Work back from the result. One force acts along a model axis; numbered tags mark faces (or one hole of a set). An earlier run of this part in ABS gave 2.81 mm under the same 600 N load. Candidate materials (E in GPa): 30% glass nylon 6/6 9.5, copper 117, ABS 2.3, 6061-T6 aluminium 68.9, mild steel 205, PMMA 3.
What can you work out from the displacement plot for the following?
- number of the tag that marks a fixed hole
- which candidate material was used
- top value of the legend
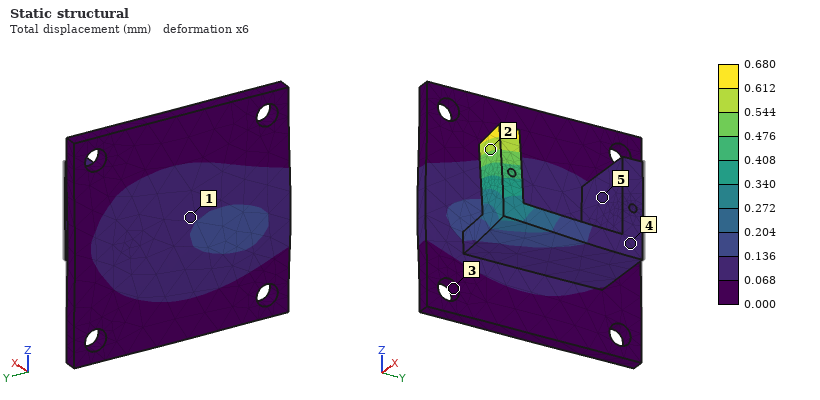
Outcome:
3
30% glass nylon 6/6
0.680 mm
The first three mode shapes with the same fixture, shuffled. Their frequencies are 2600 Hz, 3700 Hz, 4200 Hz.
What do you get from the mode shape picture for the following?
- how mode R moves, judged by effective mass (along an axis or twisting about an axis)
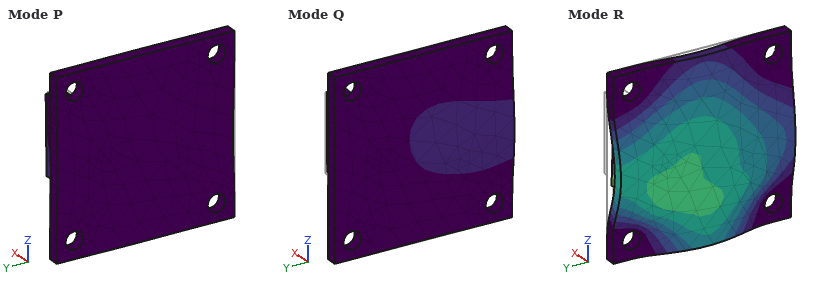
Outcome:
along X
